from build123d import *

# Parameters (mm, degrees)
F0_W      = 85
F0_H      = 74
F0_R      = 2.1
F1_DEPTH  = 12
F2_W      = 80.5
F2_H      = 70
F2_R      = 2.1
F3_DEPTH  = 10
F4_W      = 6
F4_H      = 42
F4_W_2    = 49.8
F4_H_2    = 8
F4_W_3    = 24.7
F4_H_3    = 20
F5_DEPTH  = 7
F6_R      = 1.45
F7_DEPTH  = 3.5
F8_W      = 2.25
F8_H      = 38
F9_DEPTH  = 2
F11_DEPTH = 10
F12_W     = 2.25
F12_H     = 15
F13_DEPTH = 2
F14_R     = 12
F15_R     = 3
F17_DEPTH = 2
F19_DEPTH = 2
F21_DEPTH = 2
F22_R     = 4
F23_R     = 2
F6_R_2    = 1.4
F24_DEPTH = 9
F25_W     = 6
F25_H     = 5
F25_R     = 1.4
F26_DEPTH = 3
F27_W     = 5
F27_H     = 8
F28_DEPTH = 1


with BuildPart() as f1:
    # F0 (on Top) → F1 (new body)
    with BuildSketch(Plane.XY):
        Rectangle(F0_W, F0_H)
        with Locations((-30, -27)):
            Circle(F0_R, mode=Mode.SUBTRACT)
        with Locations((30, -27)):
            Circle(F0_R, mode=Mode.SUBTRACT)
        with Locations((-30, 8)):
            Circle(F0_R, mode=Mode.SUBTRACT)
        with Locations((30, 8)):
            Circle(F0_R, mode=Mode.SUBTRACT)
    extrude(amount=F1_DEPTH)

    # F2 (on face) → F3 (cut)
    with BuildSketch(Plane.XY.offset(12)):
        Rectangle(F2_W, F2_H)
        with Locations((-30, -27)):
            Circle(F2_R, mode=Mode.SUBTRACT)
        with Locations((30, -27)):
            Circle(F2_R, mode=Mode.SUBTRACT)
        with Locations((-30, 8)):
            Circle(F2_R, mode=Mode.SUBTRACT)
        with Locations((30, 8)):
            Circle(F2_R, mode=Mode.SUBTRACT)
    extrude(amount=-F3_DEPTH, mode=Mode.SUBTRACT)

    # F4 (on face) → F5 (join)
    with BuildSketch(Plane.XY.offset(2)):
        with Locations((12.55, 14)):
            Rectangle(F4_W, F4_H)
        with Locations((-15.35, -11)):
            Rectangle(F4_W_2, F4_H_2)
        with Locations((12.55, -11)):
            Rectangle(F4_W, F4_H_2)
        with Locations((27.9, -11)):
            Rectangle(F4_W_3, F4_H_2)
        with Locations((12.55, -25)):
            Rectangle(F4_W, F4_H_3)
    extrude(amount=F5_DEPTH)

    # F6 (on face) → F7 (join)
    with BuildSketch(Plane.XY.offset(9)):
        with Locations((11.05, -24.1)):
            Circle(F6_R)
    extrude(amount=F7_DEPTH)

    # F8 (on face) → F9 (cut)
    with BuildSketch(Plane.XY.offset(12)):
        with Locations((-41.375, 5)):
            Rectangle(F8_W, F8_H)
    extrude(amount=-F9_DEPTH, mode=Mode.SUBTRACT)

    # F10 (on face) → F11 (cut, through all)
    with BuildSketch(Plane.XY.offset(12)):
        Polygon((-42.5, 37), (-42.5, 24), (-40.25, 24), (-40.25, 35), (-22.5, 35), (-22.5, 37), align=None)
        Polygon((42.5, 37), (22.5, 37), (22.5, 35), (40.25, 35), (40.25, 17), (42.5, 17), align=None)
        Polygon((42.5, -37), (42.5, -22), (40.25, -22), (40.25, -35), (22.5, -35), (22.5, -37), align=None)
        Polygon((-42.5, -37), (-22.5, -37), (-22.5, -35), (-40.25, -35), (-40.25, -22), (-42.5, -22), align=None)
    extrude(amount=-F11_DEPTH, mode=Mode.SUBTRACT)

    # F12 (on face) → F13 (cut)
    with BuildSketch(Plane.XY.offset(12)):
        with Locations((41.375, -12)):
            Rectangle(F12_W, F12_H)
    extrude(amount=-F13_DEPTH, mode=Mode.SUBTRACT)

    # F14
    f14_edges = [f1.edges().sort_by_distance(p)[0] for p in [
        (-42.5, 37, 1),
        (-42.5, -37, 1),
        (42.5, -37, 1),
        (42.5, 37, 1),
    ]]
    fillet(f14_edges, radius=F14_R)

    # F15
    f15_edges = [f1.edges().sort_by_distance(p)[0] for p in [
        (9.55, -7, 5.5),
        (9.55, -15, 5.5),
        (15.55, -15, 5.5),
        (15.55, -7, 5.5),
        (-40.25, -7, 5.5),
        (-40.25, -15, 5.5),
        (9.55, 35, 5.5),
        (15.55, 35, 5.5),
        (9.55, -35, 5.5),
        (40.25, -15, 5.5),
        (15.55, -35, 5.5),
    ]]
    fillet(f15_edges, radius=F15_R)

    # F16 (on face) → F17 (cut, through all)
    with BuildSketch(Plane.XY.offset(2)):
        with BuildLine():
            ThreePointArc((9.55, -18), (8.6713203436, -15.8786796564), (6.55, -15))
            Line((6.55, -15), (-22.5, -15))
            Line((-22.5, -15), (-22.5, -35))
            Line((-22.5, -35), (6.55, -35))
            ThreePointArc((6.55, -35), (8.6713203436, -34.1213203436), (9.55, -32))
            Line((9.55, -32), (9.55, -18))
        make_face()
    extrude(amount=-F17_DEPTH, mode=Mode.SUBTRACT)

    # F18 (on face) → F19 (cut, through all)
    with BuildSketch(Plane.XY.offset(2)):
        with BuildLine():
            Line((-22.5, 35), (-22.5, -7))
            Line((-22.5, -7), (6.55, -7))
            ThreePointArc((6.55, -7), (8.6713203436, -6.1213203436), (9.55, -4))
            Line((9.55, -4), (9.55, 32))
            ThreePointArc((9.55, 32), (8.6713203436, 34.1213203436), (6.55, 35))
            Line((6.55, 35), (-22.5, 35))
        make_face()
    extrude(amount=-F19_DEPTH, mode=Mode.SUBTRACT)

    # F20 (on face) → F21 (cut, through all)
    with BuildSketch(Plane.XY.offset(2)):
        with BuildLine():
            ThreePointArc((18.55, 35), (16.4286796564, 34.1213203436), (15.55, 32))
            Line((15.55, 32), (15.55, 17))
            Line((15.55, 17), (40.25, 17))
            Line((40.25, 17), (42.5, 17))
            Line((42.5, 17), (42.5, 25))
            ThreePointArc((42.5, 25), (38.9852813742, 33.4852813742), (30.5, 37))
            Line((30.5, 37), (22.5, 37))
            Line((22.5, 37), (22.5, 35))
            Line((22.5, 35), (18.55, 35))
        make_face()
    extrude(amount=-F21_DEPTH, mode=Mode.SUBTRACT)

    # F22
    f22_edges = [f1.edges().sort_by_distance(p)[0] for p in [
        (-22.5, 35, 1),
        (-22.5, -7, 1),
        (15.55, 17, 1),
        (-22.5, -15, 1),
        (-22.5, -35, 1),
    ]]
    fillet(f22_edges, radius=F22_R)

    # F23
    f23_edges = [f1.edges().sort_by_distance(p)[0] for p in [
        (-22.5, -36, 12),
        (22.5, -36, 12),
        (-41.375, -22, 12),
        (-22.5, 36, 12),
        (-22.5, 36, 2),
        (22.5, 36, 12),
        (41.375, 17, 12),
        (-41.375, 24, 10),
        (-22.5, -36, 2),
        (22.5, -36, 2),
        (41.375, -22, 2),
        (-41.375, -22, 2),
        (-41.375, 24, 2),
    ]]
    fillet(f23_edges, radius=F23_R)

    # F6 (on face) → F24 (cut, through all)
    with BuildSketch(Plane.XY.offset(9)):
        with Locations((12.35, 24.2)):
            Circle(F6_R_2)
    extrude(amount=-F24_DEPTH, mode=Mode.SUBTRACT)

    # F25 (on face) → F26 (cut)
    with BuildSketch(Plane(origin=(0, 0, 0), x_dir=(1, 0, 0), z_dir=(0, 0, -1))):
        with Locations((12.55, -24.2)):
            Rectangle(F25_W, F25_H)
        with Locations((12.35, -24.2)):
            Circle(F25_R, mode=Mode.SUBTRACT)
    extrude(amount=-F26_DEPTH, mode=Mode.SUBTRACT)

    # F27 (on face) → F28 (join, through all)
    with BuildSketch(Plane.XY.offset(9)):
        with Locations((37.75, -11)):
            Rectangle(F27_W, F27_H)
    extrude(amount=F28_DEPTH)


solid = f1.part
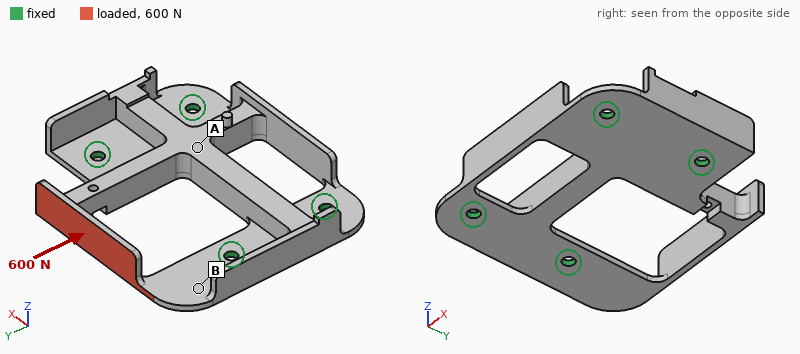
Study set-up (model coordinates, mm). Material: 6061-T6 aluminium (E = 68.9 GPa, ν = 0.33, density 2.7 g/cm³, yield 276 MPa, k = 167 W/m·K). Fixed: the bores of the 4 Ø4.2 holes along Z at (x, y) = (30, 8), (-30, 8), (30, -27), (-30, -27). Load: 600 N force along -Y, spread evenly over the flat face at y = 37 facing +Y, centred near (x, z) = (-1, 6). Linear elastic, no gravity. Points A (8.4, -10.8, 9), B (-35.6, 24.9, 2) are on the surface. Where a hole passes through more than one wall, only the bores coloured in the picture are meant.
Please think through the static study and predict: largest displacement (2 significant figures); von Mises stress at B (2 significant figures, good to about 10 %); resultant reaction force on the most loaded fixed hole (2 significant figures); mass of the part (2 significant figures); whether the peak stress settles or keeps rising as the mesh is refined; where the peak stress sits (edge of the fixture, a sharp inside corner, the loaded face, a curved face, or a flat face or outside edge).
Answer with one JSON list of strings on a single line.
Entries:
["0.26 mm", "25 MPa", "230 N", "49 g", "keeps rising", "a sharp inside corner"]
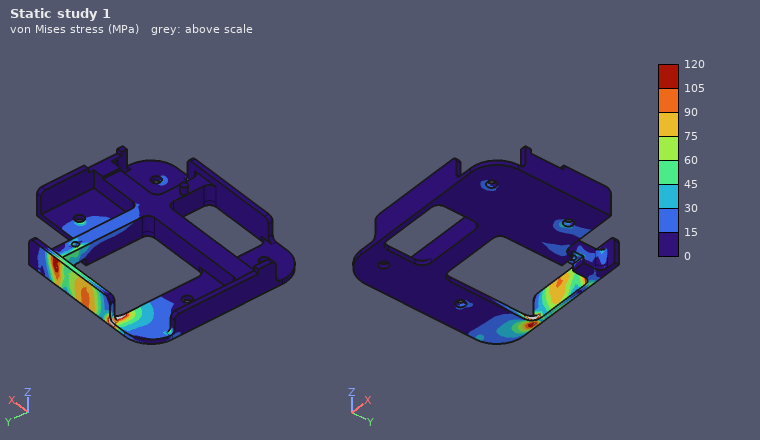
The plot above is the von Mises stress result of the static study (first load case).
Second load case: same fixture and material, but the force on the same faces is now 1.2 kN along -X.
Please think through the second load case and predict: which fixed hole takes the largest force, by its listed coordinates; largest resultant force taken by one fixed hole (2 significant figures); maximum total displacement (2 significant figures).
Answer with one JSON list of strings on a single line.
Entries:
["(-30, 8)", "1.4 kN", "0.36 mm"]
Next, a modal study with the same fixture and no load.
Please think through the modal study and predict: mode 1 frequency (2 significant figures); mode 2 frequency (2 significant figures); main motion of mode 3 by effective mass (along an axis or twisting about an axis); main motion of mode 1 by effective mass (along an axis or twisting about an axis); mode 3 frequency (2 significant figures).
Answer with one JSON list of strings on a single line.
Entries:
["2100 Hz", "3600 Hz", "along Z", "along Z", "4600 Hz"]
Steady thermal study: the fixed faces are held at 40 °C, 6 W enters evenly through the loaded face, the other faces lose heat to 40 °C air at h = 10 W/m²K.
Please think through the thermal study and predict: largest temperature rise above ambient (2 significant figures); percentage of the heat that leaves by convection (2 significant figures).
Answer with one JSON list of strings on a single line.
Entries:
["22 K", "6.8 %"]
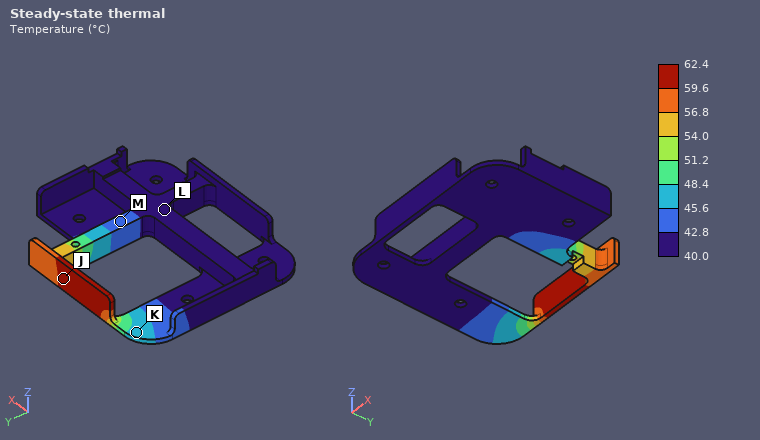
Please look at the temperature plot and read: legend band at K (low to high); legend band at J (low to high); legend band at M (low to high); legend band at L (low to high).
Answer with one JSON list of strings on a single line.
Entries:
["45.6 to 48.4 °C", "59.6 to 62.4 °C", "42.8 to 45.6 °C", "40.0 to 42.8 °C"]
